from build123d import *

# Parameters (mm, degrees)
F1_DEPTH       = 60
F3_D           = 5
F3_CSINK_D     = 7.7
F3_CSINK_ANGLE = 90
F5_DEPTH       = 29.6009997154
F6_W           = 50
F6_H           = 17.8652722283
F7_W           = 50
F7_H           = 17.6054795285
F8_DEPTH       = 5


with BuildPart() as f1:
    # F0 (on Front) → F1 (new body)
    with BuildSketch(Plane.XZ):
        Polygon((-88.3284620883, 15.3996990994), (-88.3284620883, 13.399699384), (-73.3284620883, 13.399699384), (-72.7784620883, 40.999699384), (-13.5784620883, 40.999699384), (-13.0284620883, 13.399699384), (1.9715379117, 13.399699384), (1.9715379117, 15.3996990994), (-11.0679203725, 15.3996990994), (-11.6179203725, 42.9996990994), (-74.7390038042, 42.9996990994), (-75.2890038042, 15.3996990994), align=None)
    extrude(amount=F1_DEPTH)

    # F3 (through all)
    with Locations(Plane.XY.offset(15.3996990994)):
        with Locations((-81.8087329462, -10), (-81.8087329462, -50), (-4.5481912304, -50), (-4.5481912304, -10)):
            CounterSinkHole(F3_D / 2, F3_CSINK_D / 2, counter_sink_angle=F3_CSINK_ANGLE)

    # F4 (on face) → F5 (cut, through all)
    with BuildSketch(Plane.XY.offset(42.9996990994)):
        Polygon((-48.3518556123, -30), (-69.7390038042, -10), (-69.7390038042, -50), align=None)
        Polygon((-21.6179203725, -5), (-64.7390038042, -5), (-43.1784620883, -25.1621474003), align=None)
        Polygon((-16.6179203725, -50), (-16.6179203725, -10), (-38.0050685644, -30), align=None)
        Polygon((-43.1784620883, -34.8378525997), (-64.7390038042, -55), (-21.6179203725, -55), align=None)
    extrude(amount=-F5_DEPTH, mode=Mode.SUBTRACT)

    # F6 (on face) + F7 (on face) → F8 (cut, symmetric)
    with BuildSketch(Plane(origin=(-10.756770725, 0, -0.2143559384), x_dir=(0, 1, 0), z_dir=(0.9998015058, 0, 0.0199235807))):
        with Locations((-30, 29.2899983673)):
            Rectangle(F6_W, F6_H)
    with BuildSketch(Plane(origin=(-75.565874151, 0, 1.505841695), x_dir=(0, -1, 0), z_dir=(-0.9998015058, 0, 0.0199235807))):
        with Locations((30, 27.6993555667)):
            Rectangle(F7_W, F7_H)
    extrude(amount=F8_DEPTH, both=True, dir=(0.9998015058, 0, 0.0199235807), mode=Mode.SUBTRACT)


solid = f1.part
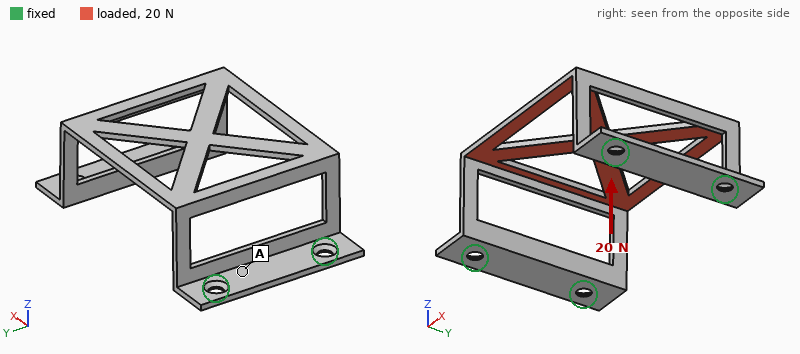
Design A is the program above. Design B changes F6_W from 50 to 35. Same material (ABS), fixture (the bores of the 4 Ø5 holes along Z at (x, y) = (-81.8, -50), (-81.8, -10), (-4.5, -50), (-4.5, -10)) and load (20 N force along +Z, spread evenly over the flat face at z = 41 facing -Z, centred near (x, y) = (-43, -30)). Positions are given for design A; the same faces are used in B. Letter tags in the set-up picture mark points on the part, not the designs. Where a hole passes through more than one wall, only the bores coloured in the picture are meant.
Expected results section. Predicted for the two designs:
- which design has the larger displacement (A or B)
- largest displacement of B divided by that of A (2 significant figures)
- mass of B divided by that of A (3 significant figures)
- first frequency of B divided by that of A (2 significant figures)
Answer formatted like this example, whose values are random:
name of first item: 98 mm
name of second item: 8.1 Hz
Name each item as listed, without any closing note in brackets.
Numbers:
which design has the larger displacement: A
largest displacement of B divided by that of A: 0.85
mass of B divided by that of A: 1.05
first frequency of B divided by that of A: 1.1
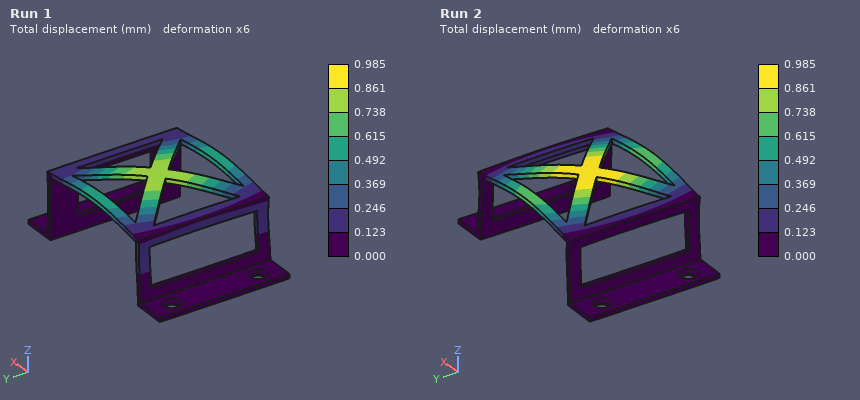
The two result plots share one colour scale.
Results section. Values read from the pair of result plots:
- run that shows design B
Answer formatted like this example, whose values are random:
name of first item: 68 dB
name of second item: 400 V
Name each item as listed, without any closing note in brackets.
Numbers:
run that shows design B: Run 1
